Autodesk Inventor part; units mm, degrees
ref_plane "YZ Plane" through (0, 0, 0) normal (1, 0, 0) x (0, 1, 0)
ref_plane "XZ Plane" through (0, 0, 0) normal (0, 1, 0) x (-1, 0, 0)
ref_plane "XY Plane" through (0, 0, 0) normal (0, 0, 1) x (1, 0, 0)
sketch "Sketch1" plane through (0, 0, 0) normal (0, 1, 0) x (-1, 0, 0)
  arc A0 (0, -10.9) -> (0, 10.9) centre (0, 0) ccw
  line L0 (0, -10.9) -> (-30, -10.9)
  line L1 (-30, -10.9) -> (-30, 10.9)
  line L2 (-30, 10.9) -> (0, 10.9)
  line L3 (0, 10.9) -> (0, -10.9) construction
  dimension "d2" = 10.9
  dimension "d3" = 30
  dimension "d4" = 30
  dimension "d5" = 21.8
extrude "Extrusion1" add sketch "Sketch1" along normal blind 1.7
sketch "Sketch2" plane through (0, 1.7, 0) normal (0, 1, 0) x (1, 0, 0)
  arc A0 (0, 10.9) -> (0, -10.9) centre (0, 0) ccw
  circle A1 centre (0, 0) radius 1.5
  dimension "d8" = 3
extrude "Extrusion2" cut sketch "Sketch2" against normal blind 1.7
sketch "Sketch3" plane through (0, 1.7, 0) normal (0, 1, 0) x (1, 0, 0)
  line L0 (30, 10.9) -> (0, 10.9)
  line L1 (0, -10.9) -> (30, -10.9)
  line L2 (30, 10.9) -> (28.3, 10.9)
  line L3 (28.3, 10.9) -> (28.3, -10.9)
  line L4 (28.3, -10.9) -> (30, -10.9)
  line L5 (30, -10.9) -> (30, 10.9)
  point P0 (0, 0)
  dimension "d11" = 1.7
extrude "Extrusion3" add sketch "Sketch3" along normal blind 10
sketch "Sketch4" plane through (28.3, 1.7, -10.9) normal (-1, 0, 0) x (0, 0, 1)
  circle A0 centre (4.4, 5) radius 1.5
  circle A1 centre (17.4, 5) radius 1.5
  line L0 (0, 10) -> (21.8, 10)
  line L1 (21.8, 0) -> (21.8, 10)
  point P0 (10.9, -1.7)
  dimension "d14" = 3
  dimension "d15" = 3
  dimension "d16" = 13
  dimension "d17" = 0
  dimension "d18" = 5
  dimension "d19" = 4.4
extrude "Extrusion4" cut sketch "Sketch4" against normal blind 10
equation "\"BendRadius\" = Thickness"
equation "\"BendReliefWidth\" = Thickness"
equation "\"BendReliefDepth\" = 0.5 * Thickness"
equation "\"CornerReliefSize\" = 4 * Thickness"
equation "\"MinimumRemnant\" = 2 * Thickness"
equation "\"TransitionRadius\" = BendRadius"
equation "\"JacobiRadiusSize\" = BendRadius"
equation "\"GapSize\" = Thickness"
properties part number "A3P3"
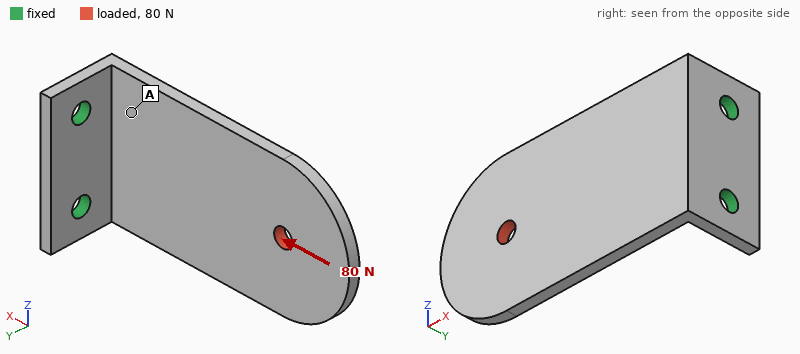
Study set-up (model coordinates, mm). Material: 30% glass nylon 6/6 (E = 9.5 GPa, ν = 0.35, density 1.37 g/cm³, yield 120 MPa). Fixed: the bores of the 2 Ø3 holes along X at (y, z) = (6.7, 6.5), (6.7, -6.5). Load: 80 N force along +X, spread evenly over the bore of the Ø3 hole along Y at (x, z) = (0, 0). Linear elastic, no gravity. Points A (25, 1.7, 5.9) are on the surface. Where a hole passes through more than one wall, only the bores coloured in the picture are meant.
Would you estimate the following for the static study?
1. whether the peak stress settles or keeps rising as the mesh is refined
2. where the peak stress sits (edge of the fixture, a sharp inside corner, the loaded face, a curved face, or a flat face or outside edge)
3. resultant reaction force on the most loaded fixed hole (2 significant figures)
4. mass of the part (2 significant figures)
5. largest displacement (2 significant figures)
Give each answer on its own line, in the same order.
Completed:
keeps rising
edge of the fixture
40 N
2.4 g
0.50 mm
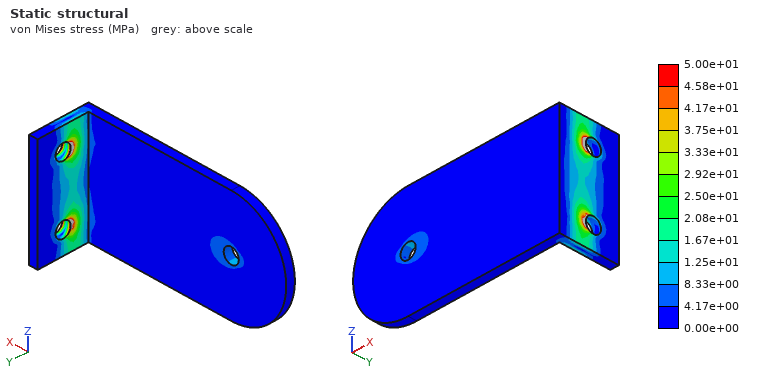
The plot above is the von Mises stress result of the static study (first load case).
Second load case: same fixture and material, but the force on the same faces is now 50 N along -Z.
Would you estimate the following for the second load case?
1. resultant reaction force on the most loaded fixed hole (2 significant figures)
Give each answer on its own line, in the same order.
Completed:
100 N
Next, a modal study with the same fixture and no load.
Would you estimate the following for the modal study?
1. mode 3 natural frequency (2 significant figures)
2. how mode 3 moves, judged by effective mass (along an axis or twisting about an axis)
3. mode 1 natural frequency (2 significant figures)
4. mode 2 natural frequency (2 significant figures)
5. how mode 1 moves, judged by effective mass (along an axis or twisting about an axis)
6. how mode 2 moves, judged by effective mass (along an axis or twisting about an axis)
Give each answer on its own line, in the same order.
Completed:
2100 Hz
along Z
430 Hz
1600 Hz
along Y
along Z
